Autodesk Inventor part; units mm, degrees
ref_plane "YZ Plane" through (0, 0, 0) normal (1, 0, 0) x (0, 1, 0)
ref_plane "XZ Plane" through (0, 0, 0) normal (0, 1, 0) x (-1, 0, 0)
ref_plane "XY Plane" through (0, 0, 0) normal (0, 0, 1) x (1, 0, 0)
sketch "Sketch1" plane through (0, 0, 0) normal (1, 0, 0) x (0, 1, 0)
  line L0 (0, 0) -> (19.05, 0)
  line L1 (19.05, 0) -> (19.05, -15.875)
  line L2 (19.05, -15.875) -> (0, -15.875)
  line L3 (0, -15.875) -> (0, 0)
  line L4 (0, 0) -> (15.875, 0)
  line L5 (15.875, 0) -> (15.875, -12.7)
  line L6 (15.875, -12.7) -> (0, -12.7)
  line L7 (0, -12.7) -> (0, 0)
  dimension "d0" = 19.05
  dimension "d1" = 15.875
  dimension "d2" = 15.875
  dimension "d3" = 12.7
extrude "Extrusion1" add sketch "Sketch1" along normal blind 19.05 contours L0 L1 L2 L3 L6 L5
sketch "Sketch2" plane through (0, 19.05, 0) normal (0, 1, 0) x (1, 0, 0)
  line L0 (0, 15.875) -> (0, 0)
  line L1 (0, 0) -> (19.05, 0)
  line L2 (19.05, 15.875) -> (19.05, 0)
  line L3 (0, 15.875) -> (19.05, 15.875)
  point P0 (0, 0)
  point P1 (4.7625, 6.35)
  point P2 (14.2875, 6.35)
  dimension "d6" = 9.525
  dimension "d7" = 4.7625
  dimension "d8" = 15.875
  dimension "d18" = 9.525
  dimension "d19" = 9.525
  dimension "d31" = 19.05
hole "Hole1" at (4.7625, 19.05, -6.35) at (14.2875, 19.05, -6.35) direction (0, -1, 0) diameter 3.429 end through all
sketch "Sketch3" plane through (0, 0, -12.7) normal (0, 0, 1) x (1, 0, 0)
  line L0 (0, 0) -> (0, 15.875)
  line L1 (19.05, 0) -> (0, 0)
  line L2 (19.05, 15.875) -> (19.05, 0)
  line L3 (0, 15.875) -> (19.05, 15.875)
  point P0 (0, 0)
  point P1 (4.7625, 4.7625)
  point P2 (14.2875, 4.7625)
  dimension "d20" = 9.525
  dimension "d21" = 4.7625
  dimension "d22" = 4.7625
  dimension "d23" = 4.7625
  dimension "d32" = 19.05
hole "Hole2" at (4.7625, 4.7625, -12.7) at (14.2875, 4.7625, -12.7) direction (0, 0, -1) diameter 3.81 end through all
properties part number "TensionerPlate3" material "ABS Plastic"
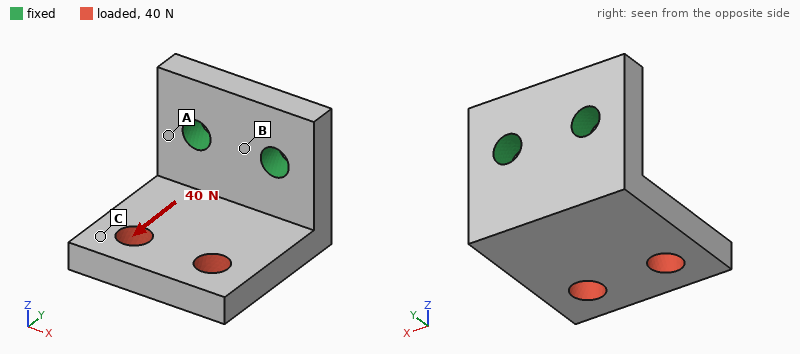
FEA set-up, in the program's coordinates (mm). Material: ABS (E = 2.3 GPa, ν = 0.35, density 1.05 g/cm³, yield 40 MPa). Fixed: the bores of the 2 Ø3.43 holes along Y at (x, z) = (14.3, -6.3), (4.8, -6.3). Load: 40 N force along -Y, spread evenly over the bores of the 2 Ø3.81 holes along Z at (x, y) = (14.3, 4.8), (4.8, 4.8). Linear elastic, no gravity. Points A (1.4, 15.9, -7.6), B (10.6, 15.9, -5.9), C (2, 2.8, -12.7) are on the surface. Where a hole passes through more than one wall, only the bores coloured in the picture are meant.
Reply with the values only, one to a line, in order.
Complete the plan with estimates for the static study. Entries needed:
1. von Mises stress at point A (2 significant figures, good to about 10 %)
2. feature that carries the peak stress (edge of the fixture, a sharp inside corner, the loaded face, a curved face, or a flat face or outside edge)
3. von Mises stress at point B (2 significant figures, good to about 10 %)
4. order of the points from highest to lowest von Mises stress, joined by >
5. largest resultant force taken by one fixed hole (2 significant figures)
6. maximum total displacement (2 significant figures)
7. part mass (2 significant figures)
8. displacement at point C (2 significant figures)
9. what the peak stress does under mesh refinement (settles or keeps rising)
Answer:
4.0 MPa
edge of the fixture
2.2 MPa
A > B > C
20 N
0.16 mm
1.9 g
0.13 mm
keeps rising
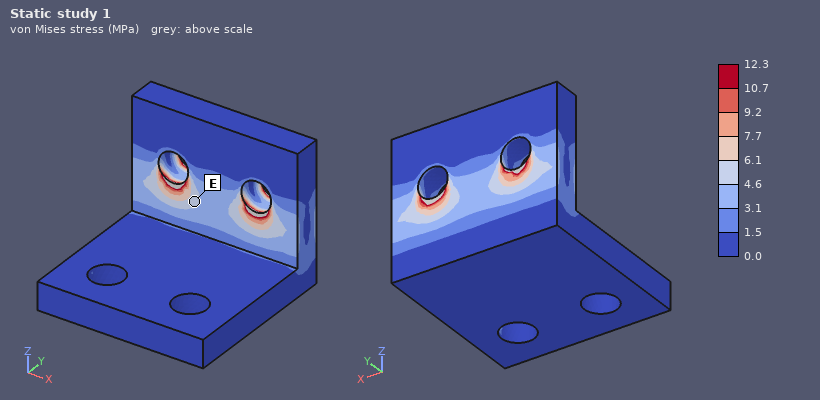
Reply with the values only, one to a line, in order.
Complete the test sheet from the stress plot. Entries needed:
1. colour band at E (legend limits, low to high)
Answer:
4.6 to 6.1 MPa
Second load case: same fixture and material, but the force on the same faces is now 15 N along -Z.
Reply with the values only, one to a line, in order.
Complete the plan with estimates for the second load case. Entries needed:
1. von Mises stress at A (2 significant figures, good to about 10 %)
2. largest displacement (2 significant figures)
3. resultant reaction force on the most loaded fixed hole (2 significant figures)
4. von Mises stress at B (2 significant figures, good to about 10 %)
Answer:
3.2 MPa
0.30 mm
8.0 N
1.7 MPa
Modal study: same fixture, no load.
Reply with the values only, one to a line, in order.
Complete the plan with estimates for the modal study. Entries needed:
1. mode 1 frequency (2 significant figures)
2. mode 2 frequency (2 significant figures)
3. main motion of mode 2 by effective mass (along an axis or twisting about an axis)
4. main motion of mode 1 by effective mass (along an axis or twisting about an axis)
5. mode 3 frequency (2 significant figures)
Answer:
1700 Hz
3200 Hz
along X
along Z
5000 Hz
